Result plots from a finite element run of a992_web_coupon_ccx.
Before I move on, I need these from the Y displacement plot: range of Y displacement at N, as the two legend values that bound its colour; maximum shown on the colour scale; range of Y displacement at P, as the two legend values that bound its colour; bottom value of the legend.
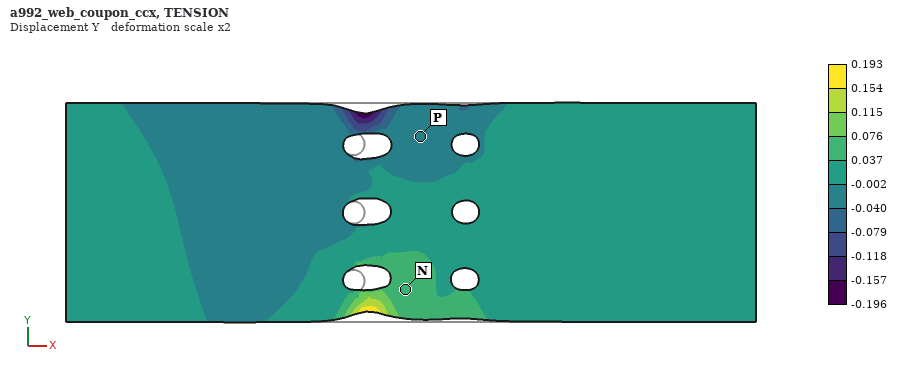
0.037 to 0.076
0.193
-0.040 to -0.002
-0.196
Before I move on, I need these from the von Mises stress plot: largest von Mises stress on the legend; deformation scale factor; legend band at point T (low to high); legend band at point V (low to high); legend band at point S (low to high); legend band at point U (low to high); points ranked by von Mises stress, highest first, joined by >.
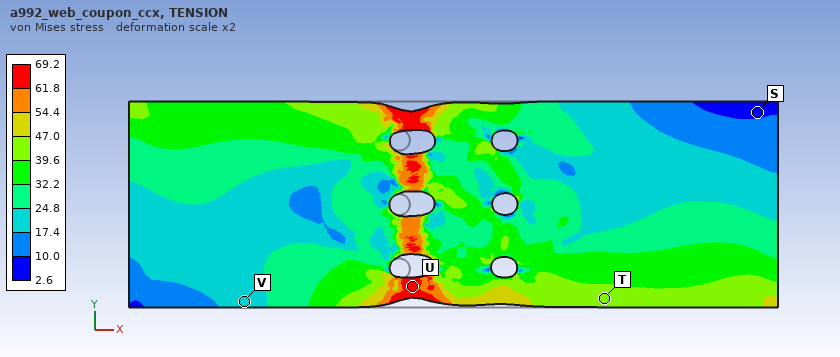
69.2
2
39.6 to 47.0
17.4 to 24.8
2.6 to 10.0
61.8 to 69.2
U > T > V > S
